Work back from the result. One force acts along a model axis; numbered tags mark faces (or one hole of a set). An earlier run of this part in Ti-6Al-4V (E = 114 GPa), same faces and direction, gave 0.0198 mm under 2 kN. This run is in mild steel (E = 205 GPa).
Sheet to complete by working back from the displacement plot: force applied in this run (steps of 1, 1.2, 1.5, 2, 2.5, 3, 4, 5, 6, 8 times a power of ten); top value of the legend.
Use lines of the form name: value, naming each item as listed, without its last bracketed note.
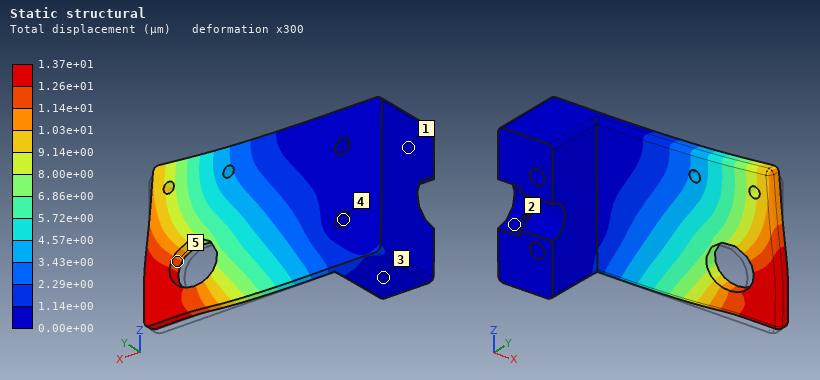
force applied in this run: 2.5 kN
top value of the legend: 1.37e+01 µm
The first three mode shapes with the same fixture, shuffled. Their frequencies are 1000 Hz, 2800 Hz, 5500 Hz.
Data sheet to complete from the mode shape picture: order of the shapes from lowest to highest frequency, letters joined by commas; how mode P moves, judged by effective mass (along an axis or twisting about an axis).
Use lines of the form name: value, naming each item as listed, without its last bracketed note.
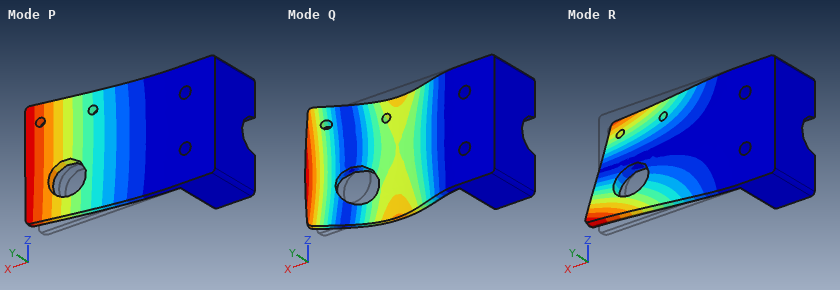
order of the shapes from lowest to highest frequency, letters joined by commas: P, R, Q
how mode P moves, judged by effective mass: along Y
